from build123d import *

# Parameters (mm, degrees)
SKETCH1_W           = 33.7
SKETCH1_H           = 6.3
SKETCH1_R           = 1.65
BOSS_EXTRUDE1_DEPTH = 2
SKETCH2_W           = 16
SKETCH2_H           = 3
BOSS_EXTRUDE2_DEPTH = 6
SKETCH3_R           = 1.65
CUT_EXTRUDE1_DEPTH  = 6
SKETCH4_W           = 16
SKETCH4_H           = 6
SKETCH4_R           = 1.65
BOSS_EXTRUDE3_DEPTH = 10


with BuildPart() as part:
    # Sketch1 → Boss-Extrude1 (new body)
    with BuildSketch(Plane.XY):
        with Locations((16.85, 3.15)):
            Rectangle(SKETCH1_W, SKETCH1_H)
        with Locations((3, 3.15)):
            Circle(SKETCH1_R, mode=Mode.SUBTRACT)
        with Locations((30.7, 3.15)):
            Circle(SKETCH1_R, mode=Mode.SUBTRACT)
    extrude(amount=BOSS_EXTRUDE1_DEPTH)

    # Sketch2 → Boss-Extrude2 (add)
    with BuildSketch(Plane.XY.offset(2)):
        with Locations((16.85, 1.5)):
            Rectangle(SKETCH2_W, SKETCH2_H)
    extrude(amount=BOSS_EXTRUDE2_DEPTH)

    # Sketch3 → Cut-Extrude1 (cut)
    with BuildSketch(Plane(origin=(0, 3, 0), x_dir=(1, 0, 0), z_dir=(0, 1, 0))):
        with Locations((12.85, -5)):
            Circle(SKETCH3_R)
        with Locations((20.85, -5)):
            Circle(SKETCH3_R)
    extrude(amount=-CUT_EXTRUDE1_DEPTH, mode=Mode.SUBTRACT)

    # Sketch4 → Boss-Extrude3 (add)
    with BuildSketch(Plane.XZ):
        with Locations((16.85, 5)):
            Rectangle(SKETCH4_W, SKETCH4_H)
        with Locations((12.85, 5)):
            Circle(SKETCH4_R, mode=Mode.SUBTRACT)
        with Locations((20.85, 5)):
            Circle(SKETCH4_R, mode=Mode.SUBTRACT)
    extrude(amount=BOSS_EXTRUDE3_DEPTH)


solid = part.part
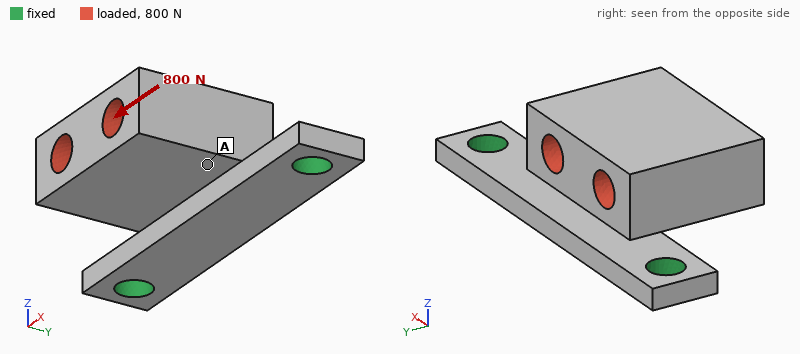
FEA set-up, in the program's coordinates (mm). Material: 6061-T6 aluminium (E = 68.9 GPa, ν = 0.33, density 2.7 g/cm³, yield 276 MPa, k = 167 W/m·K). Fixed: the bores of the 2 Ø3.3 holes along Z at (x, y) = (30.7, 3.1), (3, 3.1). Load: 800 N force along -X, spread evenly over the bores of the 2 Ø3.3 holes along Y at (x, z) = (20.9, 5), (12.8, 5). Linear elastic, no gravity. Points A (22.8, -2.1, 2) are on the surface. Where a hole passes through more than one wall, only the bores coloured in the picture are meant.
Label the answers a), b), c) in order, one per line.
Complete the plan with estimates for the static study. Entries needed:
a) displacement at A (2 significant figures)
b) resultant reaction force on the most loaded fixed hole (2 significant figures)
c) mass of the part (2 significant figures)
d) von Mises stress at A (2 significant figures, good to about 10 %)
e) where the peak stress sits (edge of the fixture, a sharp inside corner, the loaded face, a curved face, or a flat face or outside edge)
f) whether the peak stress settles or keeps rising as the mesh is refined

a) 14 µm
b) 490 N
c) 3.8 g
d) 36 MPa
e) a sharp inside corner
f) keeps rising
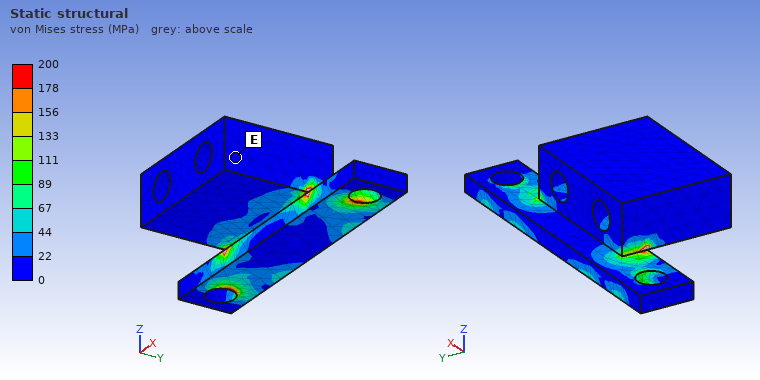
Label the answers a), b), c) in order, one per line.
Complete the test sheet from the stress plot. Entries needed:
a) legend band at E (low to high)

a) 0 to 22 MPa
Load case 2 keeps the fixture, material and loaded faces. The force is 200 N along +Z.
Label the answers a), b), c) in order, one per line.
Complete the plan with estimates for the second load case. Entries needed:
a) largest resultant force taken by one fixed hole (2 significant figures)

a) 120 N
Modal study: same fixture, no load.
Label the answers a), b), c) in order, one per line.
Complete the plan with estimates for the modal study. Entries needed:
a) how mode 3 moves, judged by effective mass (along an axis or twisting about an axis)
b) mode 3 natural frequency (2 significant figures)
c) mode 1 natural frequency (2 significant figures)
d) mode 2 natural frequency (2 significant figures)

a) along X
b) 18 kHz
c) 3800 Hz
d) 15 kHz
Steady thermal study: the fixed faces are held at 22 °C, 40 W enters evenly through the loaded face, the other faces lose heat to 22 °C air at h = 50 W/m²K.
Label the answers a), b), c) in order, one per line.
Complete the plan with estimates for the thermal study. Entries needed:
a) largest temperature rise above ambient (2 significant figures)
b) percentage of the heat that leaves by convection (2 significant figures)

a) 86 K
b) 8.7 %
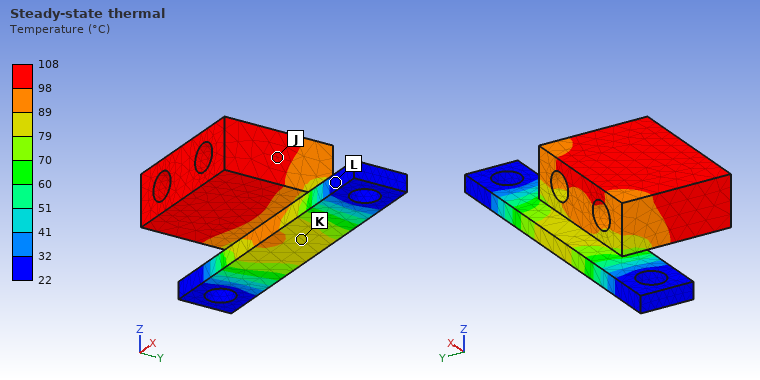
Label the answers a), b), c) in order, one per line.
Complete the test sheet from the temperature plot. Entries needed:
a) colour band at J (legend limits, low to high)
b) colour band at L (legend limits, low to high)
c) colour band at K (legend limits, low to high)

a) 98 to 108 °C
b) 22 to 32 °C
c) 79 to 89 °C
